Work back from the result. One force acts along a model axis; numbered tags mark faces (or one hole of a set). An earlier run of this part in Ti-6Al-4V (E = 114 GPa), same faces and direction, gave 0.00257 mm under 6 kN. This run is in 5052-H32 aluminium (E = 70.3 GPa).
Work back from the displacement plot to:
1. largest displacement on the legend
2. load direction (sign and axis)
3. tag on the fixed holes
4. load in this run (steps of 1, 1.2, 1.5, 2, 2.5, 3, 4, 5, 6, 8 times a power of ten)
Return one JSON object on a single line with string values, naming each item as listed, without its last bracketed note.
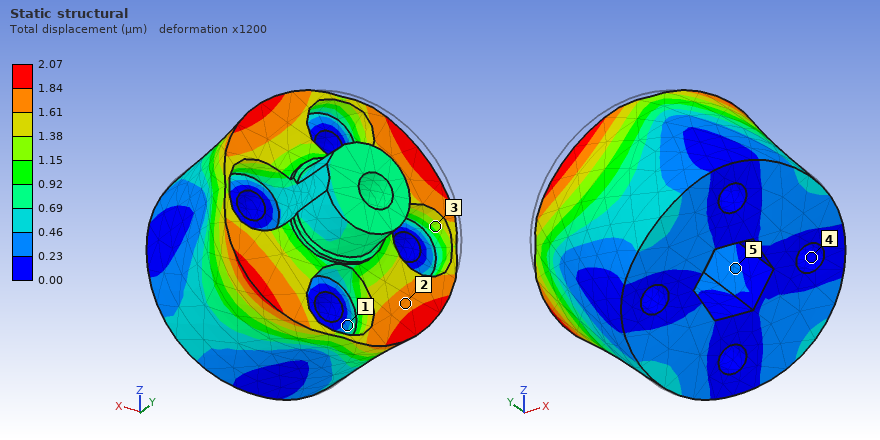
{"largest displacement on the legend": "2.07 µm", "load direction": "-Y", "tag on the fixed holes": "4", "load in this run": "3 kN"}
